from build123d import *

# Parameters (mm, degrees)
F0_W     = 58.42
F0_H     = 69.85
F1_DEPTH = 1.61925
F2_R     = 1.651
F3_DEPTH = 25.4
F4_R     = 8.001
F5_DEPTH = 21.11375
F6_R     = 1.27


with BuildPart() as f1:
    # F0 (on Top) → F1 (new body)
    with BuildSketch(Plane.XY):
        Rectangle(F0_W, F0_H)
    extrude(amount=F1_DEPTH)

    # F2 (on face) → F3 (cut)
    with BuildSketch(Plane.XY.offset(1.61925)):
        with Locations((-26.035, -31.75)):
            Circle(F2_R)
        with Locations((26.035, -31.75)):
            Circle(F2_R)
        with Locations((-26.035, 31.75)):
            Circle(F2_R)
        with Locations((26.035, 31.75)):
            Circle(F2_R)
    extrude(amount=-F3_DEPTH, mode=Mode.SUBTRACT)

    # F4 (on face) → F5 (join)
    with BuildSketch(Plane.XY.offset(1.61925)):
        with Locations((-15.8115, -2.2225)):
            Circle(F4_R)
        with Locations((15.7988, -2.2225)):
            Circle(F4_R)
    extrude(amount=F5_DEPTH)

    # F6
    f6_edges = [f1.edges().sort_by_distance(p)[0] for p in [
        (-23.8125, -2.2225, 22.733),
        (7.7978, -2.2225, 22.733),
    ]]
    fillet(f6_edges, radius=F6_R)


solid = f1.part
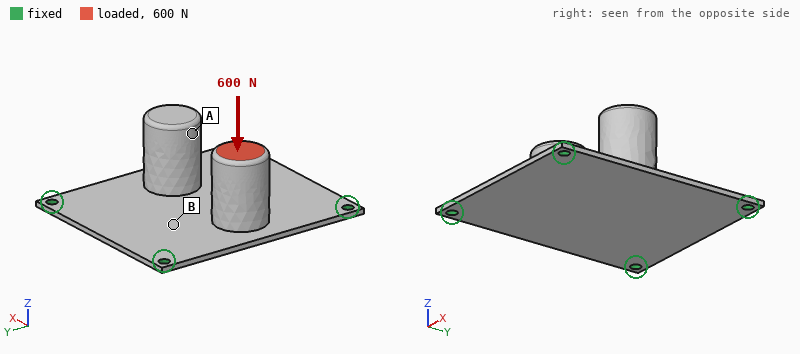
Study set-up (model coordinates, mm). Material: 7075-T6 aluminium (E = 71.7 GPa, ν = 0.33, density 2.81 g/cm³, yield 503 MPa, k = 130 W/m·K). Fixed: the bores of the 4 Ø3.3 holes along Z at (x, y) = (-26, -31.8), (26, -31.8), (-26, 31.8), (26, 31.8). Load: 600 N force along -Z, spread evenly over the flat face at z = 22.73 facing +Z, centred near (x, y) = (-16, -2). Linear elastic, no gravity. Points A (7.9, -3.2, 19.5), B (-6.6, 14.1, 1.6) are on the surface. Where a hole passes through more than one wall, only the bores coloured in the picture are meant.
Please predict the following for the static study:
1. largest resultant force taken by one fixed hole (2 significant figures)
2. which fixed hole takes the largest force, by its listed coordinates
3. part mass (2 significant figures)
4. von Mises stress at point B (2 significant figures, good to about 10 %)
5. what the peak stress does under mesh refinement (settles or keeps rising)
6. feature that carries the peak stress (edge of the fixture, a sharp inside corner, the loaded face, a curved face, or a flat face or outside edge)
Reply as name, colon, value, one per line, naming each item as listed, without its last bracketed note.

largest resultant force taken by one fixed hole: 290 N
which fixed hole takes the largest force, by its listed coordinates: (-26, -31.8)
part mass: 42 g
von Mises stress at point B: 99 MPa
what the peak stress does under mesh refinement: keeps rising
feature that carries the peak stress: edge of the fixture
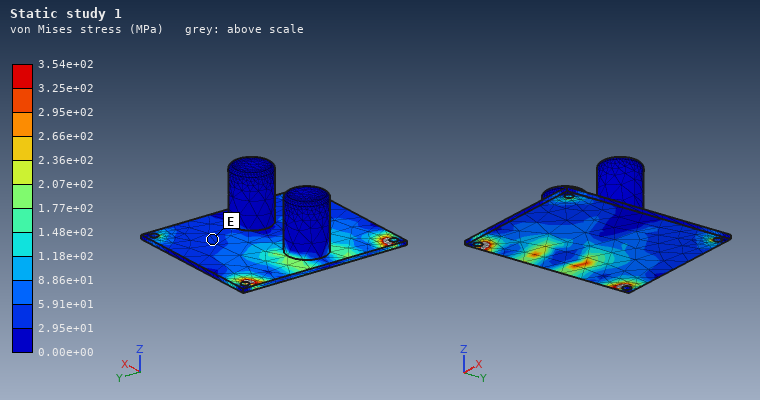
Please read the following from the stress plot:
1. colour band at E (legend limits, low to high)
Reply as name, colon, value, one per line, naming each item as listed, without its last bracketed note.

colour band at E: 2.95e+01 to 5.91e+01 MPa
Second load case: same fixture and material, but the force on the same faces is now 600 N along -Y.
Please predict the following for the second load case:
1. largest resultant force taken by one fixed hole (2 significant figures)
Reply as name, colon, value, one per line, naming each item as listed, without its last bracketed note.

largest resultant force taken by one fixed hole: 300 N
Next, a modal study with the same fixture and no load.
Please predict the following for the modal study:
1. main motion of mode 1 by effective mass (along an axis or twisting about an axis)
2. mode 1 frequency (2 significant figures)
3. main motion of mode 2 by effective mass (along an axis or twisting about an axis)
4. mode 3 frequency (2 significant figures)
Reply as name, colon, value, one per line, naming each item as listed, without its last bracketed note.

main motion of mode 1 by effective mass: along Z
mode 1 frequency: 960 Hz
main motion of mode 2 by effective mass: along X
mode 3 frequency: 1400 Hz
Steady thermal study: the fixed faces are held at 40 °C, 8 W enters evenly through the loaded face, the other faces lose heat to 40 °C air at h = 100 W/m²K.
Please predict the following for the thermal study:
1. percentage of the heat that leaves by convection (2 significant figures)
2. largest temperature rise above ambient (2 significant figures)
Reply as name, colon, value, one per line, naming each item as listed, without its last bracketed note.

percentage of the heat that leaves by convection: 60 %
largest temperature rise above ambient: 17 K
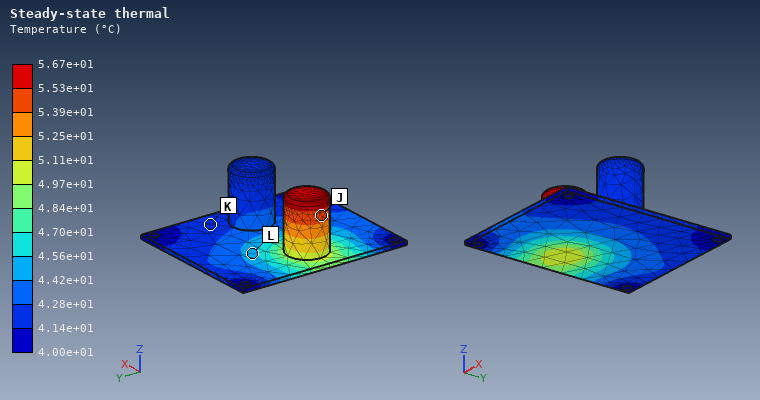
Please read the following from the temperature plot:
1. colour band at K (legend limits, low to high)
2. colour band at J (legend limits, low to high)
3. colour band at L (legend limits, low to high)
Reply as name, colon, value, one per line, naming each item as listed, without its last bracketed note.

colour band at K: 4.14e+01 to 4.28e+01 °C
colour band at J: 5.39e+01 to 5.53e+01 °C
colour band at L: 4.42e+01 to 4.56e+01 °C
